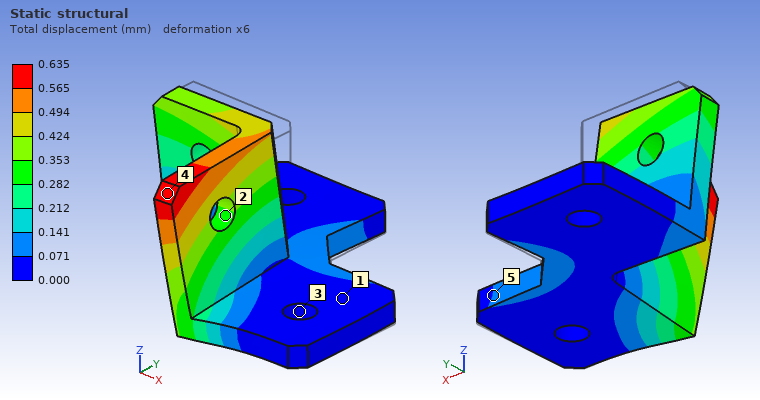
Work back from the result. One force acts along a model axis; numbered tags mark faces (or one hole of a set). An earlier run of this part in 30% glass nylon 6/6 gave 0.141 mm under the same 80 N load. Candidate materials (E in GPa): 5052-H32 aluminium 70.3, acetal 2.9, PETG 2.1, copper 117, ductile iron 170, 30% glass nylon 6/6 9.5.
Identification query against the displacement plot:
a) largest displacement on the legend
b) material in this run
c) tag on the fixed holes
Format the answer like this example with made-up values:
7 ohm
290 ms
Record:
0.635 mm
PETG
3
